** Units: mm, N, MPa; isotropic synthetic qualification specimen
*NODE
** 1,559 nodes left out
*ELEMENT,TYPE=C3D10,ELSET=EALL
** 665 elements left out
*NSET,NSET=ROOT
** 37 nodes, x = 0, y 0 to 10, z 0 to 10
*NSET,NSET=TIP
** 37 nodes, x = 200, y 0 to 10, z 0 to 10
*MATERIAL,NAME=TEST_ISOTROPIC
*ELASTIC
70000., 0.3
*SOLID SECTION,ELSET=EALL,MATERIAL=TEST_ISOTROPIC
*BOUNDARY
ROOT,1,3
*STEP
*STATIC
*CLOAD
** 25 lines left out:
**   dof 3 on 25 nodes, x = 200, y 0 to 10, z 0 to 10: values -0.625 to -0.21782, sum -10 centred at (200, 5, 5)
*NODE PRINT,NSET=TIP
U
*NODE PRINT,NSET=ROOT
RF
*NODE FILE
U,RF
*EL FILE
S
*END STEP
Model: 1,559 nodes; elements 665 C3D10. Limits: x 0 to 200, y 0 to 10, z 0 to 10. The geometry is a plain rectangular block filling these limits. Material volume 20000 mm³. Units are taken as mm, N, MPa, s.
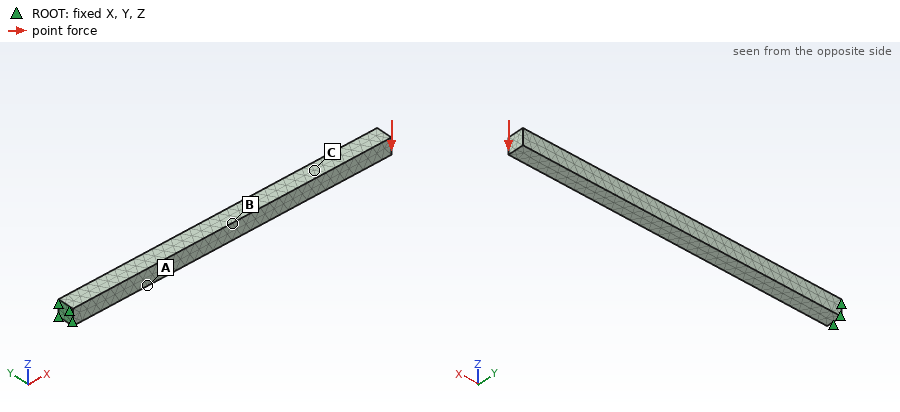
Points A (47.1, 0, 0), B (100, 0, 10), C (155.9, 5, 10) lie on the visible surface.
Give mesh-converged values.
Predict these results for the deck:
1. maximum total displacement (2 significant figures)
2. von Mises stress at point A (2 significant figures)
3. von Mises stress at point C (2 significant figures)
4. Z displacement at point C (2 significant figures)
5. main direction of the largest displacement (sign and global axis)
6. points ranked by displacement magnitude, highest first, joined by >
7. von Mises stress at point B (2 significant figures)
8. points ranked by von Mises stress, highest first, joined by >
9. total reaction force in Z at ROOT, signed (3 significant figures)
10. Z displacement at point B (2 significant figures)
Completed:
0.46 mm
9.2 MPa
2.6 MPa
-0.31 mm
-Z
C > B > A
6.0 MPa
A > B > C
10.0 N
-0.14 mm
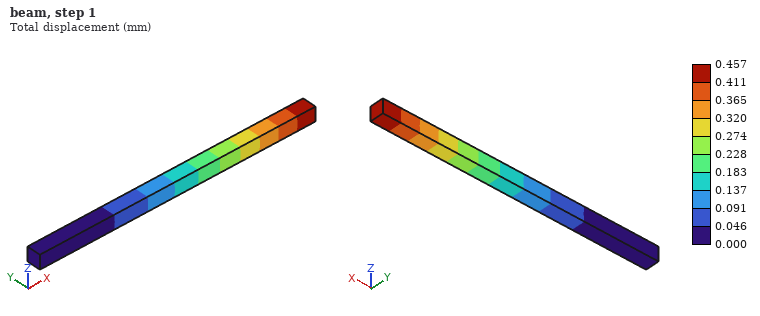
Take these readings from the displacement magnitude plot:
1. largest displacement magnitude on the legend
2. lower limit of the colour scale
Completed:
0.457 mm
0.000 mm
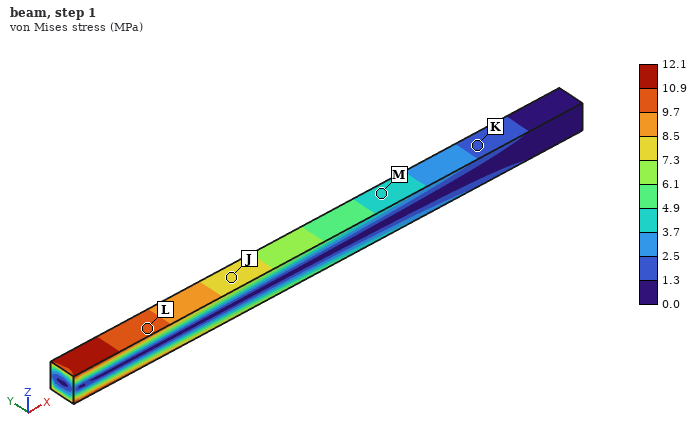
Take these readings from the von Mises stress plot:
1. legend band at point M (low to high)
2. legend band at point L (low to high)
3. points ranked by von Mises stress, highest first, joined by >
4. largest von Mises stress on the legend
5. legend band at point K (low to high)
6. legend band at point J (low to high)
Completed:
3.7 to 4.9 MPa
9.7 to 10.9 MPa
L > J > M > K
12.1 MPa
1.3 to 2.5 MPa
7.3 to 8.5 MPa
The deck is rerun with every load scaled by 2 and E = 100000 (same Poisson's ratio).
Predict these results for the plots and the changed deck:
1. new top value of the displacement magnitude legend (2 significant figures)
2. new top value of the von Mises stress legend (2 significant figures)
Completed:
0.64 mm
24 MPa
